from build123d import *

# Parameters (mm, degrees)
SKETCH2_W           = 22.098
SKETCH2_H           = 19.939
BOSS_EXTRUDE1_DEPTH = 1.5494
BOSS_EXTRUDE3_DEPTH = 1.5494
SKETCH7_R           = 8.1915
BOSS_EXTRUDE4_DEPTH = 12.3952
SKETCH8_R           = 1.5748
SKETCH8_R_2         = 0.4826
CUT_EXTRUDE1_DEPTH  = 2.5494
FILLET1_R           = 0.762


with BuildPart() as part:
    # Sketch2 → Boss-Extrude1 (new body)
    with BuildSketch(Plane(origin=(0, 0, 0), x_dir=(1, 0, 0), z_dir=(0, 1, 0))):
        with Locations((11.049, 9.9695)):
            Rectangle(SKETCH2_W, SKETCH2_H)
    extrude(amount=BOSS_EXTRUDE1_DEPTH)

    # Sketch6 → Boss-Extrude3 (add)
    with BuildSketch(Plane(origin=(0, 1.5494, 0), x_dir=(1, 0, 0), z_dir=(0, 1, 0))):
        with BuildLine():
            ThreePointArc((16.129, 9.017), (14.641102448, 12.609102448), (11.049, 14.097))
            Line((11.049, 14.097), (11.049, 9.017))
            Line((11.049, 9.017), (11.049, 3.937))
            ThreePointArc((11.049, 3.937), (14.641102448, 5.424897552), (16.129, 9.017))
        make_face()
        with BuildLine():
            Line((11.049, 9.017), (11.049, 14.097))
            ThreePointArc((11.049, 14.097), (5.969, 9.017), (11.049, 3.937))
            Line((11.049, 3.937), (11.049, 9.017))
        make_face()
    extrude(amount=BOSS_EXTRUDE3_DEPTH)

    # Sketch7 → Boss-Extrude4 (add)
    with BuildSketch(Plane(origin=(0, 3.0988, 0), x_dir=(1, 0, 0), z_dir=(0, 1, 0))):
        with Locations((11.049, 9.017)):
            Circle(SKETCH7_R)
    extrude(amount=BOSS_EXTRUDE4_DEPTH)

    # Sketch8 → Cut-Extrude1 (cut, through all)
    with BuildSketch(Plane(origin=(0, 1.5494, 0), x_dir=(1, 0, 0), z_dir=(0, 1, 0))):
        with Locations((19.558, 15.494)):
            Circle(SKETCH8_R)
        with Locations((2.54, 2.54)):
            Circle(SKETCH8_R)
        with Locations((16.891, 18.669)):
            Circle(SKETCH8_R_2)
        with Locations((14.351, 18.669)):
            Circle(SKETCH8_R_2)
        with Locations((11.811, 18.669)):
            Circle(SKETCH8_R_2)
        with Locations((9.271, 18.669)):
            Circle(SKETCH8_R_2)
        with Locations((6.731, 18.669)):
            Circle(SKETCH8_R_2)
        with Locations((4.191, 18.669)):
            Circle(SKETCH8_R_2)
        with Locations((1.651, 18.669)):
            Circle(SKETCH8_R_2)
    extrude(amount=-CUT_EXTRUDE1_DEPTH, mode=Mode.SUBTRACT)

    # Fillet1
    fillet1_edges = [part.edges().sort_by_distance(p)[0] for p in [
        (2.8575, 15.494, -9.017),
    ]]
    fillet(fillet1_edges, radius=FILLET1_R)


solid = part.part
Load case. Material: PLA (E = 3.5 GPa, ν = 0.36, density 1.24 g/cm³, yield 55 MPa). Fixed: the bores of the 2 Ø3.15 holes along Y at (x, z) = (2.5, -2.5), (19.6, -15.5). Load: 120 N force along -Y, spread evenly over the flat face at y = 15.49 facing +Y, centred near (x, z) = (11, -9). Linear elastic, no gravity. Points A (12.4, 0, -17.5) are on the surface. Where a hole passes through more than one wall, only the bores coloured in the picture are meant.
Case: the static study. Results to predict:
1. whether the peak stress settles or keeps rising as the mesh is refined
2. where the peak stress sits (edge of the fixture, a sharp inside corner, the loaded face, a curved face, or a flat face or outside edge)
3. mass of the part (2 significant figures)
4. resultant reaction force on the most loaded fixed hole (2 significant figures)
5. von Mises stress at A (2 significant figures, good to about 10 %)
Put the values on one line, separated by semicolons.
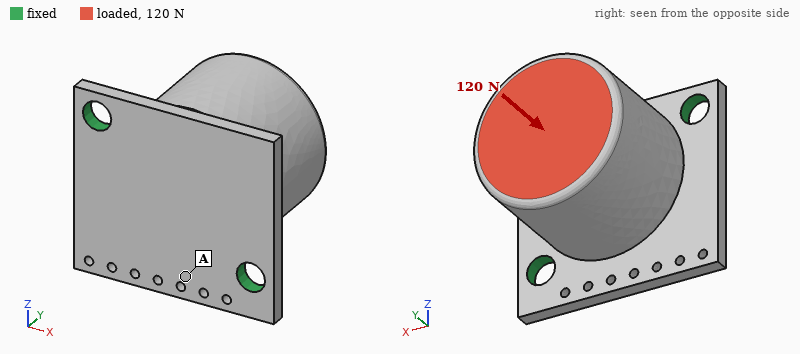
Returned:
keeps rising; edge of the fixture; 4.2 g; 64 N; 7.1 MPa
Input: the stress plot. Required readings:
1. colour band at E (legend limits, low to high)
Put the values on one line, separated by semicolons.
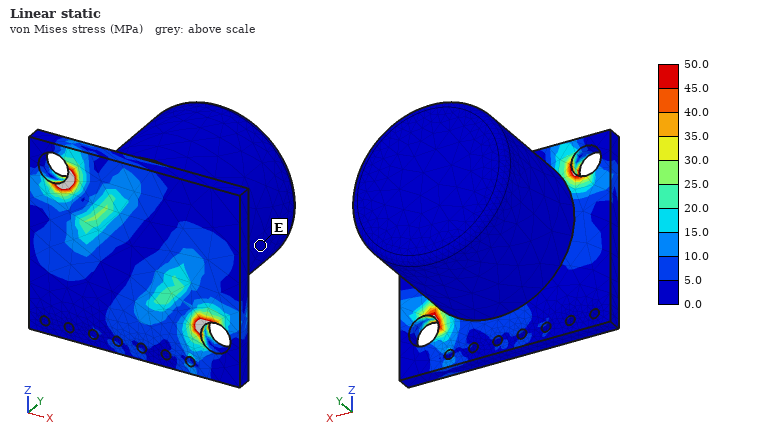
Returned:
0.0 to 5.0 MPa
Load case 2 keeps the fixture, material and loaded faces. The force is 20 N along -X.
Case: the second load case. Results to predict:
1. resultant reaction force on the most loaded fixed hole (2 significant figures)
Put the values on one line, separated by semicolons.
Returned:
18 N
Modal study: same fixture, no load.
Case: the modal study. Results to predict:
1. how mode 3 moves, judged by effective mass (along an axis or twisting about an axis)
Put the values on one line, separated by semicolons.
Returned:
along Y
